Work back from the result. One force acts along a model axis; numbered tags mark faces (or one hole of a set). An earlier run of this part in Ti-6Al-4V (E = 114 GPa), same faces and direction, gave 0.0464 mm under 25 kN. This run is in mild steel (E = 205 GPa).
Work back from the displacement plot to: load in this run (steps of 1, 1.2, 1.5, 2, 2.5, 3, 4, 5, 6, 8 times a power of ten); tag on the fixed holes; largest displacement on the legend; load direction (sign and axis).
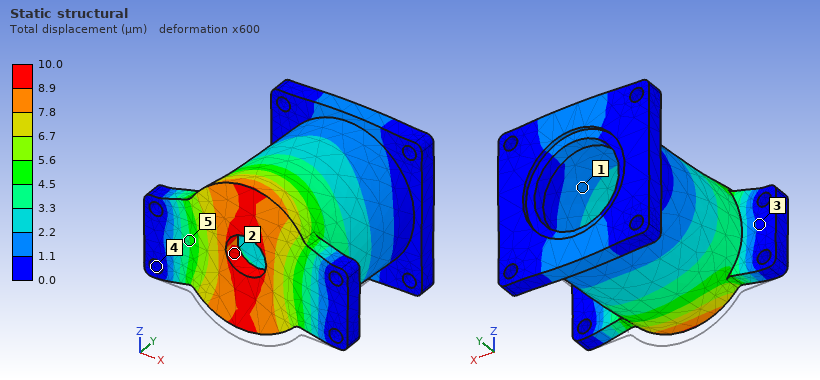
10 kN
4
10.0 µm
+Z
